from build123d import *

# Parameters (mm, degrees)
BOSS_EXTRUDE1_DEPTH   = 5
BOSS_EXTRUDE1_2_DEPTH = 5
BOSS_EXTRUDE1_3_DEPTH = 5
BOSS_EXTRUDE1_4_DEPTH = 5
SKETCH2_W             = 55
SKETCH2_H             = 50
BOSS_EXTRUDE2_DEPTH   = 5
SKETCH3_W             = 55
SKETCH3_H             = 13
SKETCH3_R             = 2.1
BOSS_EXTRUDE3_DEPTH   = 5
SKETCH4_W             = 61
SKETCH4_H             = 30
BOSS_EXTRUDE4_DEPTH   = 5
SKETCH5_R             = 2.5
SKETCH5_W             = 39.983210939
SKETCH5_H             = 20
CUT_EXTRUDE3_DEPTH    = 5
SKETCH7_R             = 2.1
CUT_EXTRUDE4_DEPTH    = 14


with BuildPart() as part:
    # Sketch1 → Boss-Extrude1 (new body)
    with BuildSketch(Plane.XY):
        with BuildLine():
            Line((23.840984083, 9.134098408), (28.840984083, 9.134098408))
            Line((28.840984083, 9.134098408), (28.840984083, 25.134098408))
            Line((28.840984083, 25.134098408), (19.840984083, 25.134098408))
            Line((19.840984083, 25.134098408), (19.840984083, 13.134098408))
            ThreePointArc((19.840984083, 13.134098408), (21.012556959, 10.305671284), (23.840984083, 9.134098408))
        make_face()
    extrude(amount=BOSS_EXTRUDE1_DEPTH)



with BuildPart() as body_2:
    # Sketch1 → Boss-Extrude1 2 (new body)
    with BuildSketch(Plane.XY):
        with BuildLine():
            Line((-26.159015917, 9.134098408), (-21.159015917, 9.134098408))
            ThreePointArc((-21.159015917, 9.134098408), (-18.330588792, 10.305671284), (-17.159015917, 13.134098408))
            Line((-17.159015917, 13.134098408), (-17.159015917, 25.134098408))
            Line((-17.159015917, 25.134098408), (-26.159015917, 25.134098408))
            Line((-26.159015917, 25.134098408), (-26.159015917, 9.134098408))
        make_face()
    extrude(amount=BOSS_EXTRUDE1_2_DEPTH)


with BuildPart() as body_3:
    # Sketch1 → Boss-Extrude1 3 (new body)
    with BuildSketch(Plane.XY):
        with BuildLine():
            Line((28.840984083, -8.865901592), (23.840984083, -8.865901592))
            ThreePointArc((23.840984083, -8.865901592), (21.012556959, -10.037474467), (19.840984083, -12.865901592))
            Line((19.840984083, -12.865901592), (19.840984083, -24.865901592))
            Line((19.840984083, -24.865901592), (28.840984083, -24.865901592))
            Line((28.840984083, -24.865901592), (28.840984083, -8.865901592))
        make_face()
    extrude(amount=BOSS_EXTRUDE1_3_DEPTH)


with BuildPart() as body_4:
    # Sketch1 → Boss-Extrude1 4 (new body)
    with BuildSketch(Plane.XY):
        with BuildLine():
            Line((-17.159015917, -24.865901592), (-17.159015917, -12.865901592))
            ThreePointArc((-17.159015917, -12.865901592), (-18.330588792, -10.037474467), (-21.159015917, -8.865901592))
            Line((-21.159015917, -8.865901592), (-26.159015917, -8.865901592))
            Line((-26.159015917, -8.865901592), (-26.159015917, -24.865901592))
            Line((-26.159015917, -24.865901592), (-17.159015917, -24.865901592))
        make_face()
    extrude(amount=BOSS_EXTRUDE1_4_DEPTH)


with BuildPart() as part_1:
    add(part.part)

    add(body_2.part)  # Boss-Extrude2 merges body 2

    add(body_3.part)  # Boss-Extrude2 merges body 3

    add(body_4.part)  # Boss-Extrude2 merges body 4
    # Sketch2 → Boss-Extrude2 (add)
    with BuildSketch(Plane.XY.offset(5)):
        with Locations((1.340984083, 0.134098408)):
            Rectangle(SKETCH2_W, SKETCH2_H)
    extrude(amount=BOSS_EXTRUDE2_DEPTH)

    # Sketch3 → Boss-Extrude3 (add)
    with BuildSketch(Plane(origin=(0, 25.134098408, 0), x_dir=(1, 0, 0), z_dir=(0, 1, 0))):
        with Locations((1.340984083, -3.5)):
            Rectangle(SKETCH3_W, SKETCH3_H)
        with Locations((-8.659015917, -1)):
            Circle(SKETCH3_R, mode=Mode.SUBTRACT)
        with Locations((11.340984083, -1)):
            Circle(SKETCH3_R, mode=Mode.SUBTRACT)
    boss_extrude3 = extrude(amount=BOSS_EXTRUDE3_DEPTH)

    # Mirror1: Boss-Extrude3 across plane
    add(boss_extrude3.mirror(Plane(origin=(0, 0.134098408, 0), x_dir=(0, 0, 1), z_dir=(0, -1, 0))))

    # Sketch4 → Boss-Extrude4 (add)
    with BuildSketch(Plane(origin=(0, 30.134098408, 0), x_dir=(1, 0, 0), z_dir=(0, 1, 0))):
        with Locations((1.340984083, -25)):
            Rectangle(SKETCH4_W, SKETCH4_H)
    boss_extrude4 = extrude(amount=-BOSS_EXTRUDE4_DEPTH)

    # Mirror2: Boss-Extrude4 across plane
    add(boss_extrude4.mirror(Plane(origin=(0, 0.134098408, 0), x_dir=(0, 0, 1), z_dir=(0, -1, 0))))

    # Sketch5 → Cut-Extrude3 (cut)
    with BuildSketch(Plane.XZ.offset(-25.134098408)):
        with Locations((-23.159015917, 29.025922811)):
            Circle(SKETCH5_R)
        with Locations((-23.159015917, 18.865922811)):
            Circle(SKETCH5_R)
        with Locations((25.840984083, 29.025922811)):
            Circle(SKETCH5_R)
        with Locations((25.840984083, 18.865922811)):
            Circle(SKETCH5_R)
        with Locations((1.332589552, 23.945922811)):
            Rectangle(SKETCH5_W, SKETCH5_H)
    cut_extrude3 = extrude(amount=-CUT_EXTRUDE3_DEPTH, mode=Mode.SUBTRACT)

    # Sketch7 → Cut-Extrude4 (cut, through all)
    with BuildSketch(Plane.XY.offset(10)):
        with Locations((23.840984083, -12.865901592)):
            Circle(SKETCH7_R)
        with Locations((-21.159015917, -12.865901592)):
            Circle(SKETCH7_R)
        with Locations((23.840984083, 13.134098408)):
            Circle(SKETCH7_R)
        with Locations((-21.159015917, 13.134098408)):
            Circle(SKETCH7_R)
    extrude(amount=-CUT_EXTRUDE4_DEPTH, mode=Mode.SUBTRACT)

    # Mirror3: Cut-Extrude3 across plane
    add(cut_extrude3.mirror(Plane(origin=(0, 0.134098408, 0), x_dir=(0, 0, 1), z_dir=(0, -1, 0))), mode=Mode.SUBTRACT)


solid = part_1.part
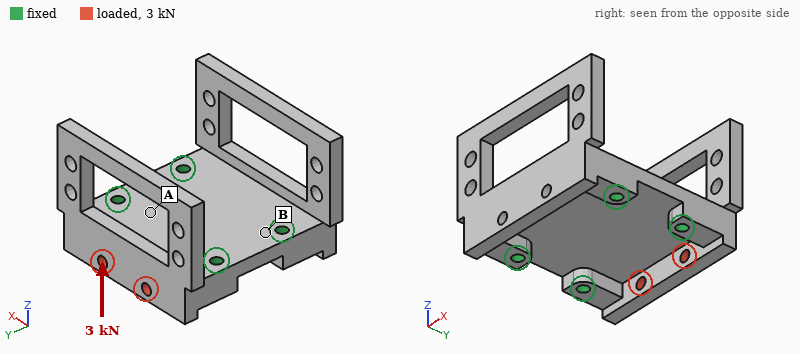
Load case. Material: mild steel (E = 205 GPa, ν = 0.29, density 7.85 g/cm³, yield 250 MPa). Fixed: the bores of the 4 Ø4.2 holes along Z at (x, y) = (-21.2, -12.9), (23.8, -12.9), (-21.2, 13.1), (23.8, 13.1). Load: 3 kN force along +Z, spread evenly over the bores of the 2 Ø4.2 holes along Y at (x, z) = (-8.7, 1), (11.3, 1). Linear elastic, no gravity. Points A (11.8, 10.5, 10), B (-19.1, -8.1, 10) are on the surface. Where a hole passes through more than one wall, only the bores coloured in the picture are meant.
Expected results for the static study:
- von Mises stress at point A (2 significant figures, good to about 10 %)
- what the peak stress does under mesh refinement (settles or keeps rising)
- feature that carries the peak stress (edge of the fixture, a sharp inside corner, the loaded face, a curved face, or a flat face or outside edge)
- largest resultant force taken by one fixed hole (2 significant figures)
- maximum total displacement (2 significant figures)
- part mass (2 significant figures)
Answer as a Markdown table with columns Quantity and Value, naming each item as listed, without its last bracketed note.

| Quantity | Value |
|---|---|
| von Mises stress at point A | 27 MPa |
| what the peak stress does under mesh refinement | keeps rising |
| feature that carries the peak stress | edge of the fixture |
| largest resultant force taken by one fixed hole | 1.6 kN |
| maximum total displacement | 30 µm |
| part mass | 250 g |
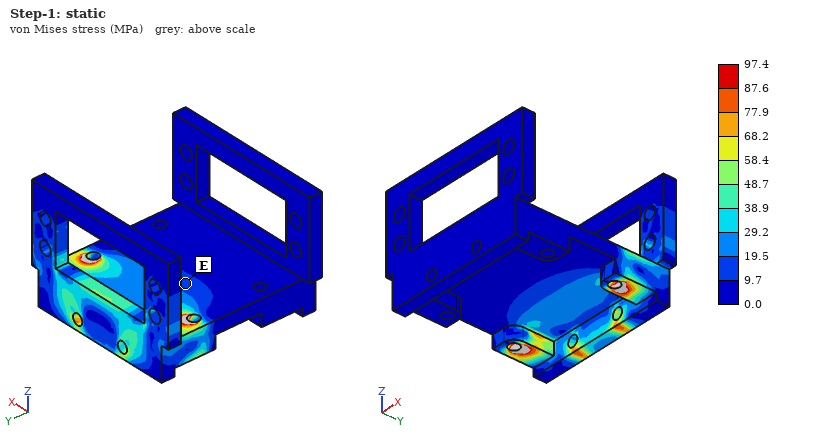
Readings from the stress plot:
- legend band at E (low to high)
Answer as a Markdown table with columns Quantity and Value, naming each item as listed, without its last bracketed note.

| Quantity | Value |
|---|---|
| legend band at E | 9.7 to 19.5 MPa |
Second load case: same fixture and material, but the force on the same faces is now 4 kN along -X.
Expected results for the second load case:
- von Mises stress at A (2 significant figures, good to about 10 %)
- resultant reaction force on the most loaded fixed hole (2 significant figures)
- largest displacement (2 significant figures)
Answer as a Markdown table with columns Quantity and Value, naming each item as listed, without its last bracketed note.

| Quantity | Value |
|---|---|
| von Mises stress at A | 9.3 MPa |
| resultant reaction force on the most loaded fixed hole | 2.2 kN |
| largest displacement | 9.5 µm |
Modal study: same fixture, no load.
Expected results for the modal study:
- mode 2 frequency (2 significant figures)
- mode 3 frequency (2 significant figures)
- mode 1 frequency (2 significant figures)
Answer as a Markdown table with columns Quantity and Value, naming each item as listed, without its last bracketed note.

| Quantity | Value |
|---|---|
| mode 2 frequency | 2200 Hz |
| mode 3 frequency | 3900 Hz |
| mode 1 frequency | 2200 Hz |
